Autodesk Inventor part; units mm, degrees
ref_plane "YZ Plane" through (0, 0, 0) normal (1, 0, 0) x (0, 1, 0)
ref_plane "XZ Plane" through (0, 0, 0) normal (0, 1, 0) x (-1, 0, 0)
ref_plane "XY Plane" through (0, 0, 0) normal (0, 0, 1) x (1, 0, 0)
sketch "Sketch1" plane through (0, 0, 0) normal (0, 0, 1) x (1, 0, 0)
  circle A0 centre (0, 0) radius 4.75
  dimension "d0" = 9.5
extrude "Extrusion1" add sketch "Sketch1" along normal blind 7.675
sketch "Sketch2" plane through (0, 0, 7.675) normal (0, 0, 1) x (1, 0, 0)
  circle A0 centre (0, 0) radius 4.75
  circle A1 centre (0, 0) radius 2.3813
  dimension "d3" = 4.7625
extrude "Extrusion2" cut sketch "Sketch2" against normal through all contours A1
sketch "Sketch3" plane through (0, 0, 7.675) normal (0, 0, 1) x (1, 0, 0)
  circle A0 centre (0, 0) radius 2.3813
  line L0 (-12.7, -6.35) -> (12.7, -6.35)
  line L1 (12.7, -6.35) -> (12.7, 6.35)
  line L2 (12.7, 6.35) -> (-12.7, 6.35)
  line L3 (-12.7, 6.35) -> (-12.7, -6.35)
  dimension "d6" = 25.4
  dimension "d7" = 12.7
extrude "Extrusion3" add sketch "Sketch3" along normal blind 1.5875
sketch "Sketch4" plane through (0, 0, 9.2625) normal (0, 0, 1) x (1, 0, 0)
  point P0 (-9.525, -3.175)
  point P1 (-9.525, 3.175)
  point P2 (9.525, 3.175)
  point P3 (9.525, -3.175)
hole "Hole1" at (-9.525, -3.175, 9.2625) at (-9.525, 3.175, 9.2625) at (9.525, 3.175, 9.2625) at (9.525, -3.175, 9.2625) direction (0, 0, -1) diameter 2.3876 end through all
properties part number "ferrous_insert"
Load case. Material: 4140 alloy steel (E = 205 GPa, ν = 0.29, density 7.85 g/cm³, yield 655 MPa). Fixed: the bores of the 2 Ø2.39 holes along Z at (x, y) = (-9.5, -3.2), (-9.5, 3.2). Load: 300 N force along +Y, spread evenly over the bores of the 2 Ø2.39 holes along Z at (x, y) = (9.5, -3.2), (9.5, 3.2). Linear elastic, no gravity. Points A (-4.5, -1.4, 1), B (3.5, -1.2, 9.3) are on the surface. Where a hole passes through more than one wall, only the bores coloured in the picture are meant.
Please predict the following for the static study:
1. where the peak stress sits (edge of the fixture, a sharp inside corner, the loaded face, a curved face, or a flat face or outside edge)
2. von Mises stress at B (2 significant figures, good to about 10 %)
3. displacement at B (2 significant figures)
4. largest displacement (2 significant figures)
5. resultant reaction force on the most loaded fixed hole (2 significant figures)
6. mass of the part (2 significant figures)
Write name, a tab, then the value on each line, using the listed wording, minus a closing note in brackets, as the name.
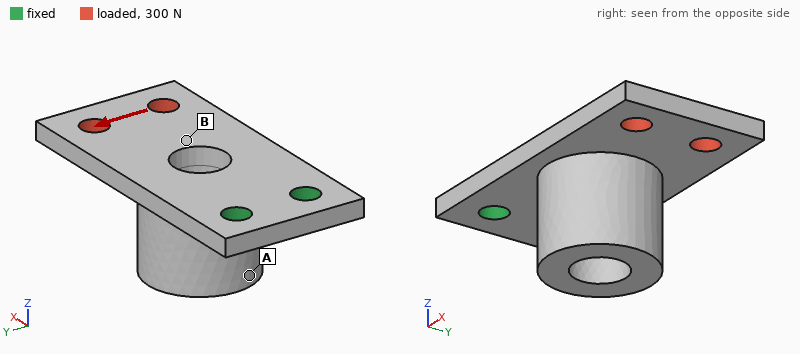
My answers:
where the peak stress sits	edge of the fixture
von Mises stress at B	46 MPa
displacement at B	12 µm
largest displacement	24 µm
resultant reaction force on the most loaded fixed hole	720 N
mass of the part	6.8 g
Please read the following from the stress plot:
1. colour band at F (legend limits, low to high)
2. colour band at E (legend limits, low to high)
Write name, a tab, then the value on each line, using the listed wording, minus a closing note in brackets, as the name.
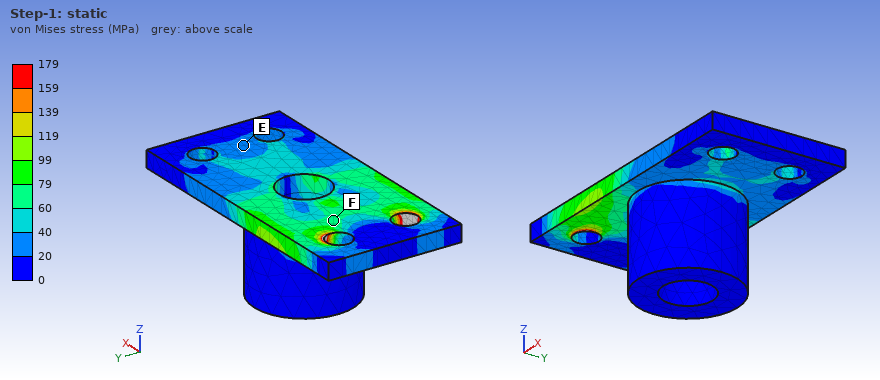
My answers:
colour band at F	60 to 79 MPa
colour band at E	20 to 40 MPa
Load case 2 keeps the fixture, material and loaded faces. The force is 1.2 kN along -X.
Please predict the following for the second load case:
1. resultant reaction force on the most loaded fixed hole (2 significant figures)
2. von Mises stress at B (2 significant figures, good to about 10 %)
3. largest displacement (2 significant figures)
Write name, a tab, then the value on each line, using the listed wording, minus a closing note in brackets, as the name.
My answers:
resultant reaction force on the most loaded fixed hole	600 N
von Mises stress at B	55 MPa
largest displacement	15 µm
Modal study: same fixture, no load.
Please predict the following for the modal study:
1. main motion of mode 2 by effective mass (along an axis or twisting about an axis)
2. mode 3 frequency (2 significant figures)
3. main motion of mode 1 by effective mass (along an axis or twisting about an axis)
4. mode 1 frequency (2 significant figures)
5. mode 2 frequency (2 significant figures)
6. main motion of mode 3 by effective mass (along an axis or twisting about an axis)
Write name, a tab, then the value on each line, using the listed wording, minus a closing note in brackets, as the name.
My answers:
main motion of mode 2 by effective mass	along Y
mode 3 frequency	15 kHz
main motion of mode 1 by effective mass	along Z
mode 1 frequency	2700 Hz
mode 2 frequency	9200 Hz
main motion of mode 3 by effective mass	along Y
